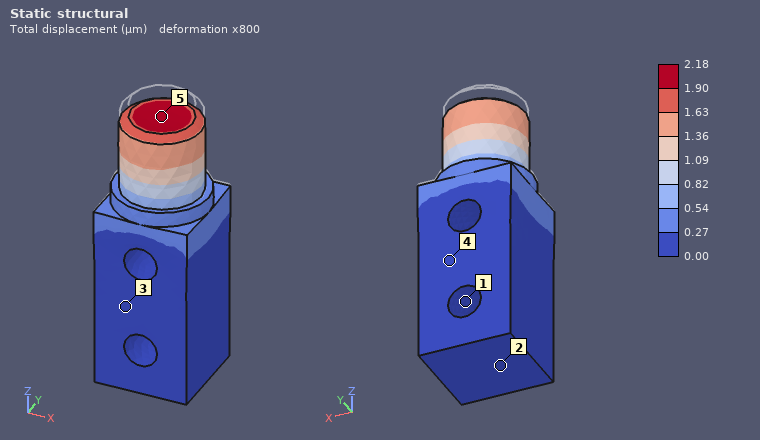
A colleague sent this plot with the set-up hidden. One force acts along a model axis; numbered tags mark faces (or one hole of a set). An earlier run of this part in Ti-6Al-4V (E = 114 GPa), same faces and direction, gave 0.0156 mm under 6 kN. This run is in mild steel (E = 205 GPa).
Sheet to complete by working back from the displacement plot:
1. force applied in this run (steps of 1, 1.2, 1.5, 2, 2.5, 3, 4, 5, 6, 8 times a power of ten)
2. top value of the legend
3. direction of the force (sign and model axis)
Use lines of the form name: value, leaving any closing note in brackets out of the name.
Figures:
force applied in this run: 1.5 kN
top value of the legend: 2.18 µm
direction of the force: -Z
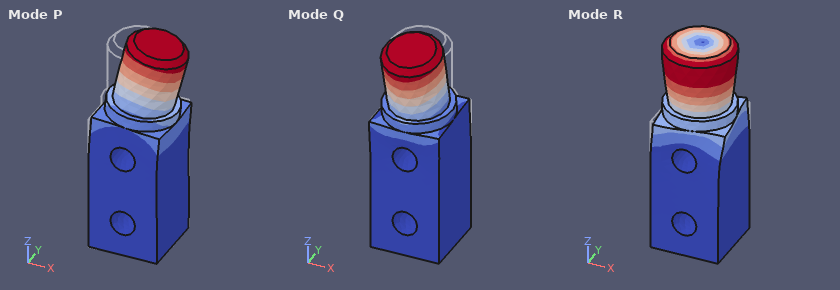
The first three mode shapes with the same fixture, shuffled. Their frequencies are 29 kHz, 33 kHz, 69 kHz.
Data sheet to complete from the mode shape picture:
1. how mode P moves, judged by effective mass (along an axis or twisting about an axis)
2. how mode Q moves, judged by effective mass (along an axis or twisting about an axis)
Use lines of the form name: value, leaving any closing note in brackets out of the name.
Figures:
how mode P moves, judged by effective mass: along X
how mode Q moves, judged by effective mass: along Y
